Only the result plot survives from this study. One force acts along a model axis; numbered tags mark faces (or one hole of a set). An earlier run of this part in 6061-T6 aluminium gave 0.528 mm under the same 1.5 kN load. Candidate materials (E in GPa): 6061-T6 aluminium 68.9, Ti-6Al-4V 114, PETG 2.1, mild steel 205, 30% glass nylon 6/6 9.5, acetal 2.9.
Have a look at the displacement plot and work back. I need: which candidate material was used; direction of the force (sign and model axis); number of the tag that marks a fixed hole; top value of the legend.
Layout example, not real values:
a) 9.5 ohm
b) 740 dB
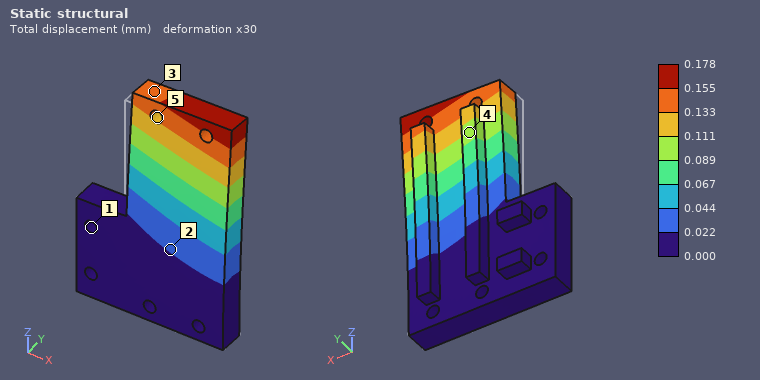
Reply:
a) mild steel
b) +Y
c) 1
d) 0.178 mm
